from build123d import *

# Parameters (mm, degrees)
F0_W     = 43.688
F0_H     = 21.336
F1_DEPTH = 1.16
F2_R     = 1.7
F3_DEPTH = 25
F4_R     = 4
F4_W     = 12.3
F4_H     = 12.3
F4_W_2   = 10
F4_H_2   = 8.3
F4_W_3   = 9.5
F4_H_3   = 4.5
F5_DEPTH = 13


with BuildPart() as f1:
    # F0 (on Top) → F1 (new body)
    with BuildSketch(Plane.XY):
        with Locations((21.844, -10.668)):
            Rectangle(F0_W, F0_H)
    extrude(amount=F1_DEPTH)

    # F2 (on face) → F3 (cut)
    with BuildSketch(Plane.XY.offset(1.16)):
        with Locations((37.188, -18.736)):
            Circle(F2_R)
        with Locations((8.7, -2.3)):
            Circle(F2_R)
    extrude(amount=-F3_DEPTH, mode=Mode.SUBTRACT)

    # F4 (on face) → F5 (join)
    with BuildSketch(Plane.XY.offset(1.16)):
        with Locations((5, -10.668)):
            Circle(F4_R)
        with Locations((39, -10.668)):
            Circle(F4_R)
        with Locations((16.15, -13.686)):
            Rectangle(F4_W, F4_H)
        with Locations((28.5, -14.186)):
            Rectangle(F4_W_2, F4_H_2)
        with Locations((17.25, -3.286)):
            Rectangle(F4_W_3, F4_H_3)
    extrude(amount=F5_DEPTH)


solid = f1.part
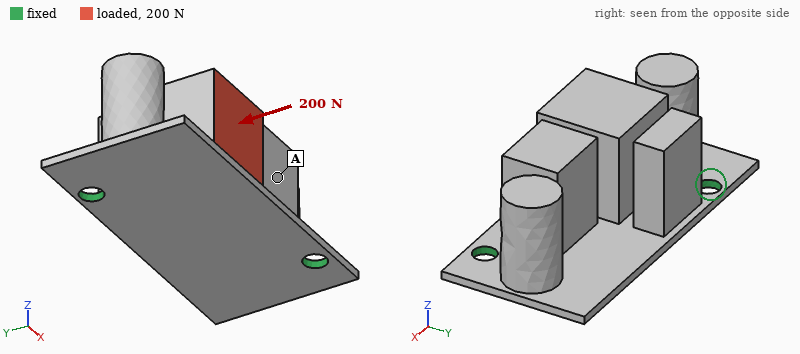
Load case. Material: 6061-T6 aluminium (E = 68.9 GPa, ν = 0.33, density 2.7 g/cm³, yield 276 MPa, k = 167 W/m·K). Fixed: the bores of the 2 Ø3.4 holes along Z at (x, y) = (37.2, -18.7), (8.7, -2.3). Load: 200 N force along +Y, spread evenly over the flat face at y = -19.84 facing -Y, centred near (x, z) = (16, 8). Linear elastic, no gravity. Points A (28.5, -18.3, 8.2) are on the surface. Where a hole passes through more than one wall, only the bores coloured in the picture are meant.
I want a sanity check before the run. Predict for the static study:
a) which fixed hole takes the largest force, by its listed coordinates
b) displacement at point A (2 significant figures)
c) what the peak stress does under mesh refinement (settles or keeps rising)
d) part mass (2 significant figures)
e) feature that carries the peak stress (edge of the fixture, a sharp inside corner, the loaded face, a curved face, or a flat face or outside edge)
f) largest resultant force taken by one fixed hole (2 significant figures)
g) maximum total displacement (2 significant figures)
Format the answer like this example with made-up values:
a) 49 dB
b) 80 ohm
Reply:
a) (8.7, -2.3)
b) 0.089 mm
c) keeps rising
d) 16 g
e) edge of the fixture
f) 140 N
g) 0.22 mm
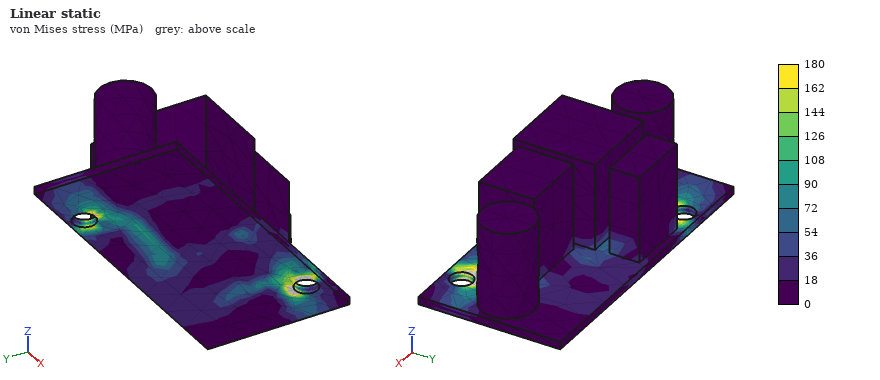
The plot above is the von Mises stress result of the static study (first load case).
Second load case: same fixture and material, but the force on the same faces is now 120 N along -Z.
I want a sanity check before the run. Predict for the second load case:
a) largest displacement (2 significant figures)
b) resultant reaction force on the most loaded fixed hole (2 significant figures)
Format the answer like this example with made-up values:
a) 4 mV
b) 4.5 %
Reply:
a) 0.22 mm
b) 82 N
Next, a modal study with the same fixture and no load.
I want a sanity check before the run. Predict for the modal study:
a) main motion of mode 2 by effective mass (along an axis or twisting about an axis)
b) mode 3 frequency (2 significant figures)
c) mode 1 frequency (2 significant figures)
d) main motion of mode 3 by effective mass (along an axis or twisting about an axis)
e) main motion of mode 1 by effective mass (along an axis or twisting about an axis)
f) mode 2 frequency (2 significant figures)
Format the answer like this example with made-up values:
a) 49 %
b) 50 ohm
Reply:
a) along Z
b) 3200 Hz
c) 1500 Hz
d) along Z
e) along Y
f) 2700 Hz
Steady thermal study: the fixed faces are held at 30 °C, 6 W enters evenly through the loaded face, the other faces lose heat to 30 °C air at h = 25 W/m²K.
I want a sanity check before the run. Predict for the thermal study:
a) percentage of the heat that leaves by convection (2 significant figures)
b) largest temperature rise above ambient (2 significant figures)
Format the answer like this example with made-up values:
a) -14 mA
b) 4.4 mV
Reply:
a) 9.5 %
b) 11 K
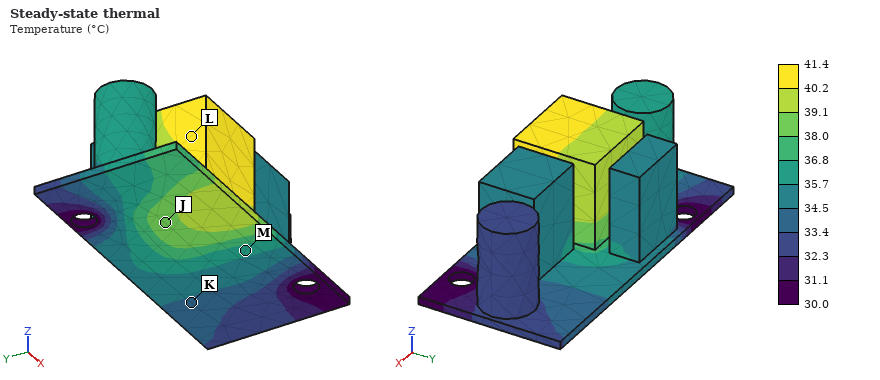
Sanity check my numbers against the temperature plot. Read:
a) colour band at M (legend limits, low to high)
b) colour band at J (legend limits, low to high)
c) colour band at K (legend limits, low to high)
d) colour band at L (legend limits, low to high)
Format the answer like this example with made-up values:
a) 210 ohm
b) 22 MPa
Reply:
a) 35.7 to 36.8 °C
b) 38.0 to 39.1 °C
c) 33.4 to 34.5 °C
d) 40.2 to 41.4 °C
